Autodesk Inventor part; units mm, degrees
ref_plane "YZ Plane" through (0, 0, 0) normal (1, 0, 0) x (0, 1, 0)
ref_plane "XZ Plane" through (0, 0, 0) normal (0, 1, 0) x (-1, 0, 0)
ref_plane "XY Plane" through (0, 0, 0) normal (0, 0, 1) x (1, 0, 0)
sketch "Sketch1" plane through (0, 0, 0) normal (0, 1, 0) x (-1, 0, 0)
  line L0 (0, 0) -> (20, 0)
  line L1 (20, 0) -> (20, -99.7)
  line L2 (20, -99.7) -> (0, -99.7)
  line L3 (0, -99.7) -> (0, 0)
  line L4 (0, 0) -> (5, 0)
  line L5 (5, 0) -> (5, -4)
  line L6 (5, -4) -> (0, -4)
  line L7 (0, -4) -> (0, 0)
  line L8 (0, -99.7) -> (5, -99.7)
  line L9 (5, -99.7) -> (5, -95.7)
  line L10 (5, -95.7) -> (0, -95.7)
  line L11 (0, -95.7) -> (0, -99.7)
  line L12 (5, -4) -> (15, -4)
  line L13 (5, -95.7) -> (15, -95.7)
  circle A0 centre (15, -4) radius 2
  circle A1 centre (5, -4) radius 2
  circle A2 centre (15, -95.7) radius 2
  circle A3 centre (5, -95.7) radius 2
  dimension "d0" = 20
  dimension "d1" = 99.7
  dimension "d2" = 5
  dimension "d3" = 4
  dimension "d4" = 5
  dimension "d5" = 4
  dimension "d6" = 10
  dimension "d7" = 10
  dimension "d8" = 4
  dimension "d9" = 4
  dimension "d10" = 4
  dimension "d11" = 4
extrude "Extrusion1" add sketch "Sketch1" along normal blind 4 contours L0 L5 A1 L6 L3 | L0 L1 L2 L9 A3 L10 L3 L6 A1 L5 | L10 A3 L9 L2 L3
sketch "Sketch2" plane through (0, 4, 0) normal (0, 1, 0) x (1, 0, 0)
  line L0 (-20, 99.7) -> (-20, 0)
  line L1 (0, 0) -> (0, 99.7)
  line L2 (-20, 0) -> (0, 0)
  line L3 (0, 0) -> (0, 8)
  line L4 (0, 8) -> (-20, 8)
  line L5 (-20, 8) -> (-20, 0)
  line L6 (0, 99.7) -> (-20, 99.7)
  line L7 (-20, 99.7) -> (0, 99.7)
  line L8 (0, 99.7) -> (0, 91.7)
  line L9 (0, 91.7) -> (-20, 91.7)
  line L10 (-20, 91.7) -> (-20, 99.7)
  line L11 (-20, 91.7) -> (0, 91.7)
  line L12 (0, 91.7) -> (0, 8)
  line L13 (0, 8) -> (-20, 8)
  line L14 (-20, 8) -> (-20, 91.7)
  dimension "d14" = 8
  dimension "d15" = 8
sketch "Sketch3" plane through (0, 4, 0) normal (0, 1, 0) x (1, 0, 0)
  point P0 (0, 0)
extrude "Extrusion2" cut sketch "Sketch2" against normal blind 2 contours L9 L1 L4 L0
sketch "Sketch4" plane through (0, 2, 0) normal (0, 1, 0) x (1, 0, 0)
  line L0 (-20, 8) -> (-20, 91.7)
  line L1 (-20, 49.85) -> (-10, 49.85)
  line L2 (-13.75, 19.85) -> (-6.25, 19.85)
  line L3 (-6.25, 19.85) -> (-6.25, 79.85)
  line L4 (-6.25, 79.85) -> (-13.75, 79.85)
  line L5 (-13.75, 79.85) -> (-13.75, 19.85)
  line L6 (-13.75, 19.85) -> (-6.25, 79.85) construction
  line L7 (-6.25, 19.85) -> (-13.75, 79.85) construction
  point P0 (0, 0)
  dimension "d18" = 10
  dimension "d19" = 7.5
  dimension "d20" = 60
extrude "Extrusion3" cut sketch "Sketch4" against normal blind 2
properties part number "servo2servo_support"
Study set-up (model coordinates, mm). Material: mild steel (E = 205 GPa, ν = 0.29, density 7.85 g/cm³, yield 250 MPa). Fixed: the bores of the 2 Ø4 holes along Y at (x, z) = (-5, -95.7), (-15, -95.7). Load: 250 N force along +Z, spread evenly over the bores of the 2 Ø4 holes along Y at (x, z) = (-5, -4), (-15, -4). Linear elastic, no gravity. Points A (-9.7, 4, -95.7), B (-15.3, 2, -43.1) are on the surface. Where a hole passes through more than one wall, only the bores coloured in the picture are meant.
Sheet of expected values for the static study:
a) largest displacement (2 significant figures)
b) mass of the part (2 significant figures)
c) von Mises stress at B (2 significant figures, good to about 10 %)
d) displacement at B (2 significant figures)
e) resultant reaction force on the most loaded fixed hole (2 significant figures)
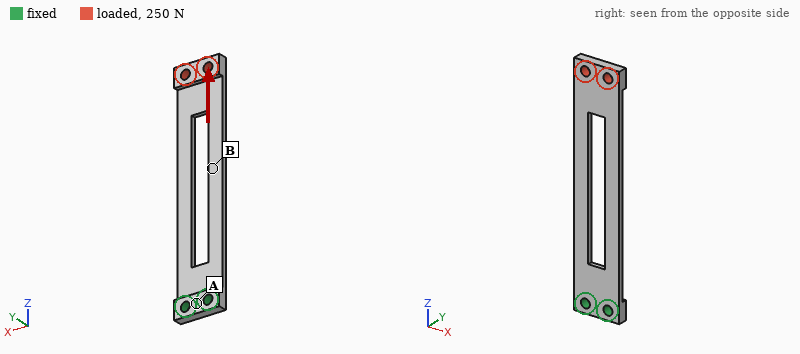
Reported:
0.56 mm
28 g
40 MPa
0.15 mm
130 N
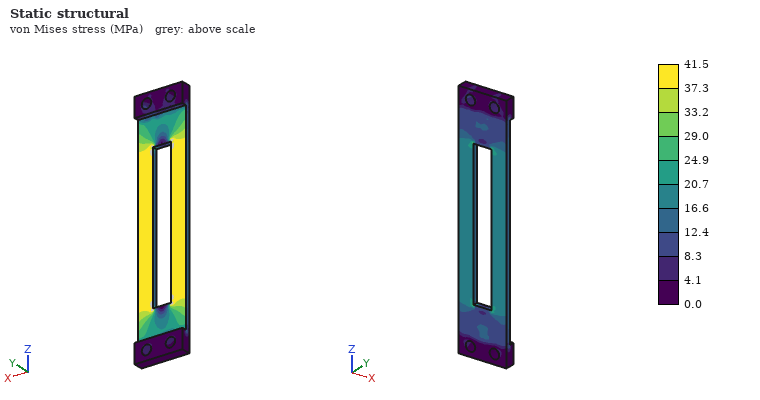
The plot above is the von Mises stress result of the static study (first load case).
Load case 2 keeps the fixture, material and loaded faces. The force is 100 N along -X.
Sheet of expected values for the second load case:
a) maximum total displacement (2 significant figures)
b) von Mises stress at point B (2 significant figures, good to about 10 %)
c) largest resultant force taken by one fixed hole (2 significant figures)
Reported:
0.26 mm
38 MPa
700 N
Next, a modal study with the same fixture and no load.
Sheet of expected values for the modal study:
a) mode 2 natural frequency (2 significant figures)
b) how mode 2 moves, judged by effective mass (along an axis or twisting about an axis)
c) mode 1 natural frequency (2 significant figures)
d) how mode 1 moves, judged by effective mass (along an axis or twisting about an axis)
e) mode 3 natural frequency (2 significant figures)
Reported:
990 Hz
along X
160 Hz
along Y
1100 Hz
